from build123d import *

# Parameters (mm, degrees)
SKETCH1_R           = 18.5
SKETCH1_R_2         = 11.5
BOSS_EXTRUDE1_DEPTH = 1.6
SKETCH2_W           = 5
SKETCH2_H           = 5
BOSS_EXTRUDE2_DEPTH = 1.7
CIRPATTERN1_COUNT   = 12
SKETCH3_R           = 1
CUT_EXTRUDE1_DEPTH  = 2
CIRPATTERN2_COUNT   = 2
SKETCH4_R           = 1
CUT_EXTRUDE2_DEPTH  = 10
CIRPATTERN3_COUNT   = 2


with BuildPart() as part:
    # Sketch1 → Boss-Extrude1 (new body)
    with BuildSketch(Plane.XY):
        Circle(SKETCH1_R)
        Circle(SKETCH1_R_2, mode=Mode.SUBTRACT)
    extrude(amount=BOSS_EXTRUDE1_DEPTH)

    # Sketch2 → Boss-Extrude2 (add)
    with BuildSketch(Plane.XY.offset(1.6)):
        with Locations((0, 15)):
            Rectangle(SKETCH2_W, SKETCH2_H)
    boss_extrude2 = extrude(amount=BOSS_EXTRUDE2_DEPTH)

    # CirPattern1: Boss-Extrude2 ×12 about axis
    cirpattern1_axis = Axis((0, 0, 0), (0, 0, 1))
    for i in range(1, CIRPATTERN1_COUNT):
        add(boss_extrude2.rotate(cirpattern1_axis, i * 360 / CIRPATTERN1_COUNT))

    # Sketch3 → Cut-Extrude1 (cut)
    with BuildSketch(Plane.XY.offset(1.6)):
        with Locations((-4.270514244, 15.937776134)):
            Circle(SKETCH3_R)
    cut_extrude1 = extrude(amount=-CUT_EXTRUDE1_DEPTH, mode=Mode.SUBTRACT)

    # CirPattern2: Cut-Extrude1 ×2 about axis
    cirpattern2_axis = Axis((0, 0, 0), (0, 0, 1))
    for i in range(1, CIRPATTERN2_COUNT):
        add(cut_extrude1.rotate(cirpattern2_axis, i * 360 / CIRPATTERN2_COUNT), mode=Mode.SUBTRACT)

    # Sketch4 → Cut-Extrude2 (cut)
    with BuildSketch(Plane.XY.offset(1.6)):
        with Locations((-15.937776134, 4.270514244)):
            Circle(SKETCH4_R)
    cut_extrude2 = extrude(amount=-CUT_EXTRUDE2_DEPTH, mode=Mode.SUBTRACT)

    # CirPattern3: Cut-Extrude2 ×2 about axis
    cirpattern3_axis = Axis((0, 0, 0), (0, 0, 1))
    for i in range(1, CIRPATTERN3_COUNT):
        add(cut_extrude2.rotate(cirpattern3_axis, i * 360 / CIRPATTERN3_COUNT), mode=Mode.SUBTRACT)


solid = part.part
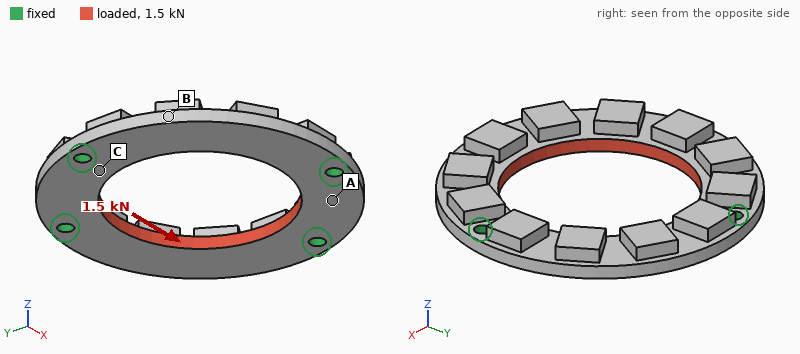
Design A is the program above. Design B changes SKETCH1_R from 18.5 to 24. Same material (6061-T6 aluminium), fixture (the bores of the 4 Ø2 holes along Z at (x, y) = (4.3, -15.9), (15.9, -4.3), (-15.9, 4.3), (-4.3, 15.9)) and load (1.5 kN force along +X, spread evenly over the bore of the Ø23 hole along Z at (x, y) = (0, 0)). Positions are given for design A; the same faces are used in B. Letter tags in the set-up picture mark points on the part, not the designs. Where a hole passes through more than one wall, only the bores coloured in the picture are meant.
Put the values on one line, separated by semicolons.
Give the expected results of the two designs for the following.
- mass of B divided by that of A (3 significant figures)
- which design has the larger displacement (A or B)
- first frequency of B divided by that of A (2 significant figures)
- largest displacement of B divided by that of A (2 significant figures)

1.76; A; 0.71; 0.64
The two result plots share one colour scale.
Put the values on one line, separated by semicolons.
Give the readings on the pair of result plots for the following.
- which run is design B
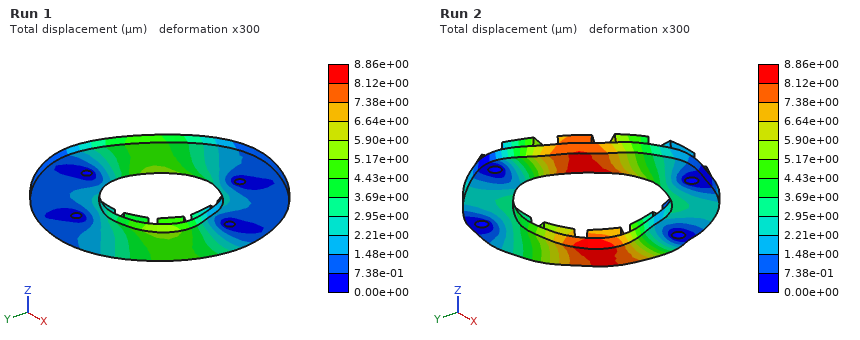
Run 1
